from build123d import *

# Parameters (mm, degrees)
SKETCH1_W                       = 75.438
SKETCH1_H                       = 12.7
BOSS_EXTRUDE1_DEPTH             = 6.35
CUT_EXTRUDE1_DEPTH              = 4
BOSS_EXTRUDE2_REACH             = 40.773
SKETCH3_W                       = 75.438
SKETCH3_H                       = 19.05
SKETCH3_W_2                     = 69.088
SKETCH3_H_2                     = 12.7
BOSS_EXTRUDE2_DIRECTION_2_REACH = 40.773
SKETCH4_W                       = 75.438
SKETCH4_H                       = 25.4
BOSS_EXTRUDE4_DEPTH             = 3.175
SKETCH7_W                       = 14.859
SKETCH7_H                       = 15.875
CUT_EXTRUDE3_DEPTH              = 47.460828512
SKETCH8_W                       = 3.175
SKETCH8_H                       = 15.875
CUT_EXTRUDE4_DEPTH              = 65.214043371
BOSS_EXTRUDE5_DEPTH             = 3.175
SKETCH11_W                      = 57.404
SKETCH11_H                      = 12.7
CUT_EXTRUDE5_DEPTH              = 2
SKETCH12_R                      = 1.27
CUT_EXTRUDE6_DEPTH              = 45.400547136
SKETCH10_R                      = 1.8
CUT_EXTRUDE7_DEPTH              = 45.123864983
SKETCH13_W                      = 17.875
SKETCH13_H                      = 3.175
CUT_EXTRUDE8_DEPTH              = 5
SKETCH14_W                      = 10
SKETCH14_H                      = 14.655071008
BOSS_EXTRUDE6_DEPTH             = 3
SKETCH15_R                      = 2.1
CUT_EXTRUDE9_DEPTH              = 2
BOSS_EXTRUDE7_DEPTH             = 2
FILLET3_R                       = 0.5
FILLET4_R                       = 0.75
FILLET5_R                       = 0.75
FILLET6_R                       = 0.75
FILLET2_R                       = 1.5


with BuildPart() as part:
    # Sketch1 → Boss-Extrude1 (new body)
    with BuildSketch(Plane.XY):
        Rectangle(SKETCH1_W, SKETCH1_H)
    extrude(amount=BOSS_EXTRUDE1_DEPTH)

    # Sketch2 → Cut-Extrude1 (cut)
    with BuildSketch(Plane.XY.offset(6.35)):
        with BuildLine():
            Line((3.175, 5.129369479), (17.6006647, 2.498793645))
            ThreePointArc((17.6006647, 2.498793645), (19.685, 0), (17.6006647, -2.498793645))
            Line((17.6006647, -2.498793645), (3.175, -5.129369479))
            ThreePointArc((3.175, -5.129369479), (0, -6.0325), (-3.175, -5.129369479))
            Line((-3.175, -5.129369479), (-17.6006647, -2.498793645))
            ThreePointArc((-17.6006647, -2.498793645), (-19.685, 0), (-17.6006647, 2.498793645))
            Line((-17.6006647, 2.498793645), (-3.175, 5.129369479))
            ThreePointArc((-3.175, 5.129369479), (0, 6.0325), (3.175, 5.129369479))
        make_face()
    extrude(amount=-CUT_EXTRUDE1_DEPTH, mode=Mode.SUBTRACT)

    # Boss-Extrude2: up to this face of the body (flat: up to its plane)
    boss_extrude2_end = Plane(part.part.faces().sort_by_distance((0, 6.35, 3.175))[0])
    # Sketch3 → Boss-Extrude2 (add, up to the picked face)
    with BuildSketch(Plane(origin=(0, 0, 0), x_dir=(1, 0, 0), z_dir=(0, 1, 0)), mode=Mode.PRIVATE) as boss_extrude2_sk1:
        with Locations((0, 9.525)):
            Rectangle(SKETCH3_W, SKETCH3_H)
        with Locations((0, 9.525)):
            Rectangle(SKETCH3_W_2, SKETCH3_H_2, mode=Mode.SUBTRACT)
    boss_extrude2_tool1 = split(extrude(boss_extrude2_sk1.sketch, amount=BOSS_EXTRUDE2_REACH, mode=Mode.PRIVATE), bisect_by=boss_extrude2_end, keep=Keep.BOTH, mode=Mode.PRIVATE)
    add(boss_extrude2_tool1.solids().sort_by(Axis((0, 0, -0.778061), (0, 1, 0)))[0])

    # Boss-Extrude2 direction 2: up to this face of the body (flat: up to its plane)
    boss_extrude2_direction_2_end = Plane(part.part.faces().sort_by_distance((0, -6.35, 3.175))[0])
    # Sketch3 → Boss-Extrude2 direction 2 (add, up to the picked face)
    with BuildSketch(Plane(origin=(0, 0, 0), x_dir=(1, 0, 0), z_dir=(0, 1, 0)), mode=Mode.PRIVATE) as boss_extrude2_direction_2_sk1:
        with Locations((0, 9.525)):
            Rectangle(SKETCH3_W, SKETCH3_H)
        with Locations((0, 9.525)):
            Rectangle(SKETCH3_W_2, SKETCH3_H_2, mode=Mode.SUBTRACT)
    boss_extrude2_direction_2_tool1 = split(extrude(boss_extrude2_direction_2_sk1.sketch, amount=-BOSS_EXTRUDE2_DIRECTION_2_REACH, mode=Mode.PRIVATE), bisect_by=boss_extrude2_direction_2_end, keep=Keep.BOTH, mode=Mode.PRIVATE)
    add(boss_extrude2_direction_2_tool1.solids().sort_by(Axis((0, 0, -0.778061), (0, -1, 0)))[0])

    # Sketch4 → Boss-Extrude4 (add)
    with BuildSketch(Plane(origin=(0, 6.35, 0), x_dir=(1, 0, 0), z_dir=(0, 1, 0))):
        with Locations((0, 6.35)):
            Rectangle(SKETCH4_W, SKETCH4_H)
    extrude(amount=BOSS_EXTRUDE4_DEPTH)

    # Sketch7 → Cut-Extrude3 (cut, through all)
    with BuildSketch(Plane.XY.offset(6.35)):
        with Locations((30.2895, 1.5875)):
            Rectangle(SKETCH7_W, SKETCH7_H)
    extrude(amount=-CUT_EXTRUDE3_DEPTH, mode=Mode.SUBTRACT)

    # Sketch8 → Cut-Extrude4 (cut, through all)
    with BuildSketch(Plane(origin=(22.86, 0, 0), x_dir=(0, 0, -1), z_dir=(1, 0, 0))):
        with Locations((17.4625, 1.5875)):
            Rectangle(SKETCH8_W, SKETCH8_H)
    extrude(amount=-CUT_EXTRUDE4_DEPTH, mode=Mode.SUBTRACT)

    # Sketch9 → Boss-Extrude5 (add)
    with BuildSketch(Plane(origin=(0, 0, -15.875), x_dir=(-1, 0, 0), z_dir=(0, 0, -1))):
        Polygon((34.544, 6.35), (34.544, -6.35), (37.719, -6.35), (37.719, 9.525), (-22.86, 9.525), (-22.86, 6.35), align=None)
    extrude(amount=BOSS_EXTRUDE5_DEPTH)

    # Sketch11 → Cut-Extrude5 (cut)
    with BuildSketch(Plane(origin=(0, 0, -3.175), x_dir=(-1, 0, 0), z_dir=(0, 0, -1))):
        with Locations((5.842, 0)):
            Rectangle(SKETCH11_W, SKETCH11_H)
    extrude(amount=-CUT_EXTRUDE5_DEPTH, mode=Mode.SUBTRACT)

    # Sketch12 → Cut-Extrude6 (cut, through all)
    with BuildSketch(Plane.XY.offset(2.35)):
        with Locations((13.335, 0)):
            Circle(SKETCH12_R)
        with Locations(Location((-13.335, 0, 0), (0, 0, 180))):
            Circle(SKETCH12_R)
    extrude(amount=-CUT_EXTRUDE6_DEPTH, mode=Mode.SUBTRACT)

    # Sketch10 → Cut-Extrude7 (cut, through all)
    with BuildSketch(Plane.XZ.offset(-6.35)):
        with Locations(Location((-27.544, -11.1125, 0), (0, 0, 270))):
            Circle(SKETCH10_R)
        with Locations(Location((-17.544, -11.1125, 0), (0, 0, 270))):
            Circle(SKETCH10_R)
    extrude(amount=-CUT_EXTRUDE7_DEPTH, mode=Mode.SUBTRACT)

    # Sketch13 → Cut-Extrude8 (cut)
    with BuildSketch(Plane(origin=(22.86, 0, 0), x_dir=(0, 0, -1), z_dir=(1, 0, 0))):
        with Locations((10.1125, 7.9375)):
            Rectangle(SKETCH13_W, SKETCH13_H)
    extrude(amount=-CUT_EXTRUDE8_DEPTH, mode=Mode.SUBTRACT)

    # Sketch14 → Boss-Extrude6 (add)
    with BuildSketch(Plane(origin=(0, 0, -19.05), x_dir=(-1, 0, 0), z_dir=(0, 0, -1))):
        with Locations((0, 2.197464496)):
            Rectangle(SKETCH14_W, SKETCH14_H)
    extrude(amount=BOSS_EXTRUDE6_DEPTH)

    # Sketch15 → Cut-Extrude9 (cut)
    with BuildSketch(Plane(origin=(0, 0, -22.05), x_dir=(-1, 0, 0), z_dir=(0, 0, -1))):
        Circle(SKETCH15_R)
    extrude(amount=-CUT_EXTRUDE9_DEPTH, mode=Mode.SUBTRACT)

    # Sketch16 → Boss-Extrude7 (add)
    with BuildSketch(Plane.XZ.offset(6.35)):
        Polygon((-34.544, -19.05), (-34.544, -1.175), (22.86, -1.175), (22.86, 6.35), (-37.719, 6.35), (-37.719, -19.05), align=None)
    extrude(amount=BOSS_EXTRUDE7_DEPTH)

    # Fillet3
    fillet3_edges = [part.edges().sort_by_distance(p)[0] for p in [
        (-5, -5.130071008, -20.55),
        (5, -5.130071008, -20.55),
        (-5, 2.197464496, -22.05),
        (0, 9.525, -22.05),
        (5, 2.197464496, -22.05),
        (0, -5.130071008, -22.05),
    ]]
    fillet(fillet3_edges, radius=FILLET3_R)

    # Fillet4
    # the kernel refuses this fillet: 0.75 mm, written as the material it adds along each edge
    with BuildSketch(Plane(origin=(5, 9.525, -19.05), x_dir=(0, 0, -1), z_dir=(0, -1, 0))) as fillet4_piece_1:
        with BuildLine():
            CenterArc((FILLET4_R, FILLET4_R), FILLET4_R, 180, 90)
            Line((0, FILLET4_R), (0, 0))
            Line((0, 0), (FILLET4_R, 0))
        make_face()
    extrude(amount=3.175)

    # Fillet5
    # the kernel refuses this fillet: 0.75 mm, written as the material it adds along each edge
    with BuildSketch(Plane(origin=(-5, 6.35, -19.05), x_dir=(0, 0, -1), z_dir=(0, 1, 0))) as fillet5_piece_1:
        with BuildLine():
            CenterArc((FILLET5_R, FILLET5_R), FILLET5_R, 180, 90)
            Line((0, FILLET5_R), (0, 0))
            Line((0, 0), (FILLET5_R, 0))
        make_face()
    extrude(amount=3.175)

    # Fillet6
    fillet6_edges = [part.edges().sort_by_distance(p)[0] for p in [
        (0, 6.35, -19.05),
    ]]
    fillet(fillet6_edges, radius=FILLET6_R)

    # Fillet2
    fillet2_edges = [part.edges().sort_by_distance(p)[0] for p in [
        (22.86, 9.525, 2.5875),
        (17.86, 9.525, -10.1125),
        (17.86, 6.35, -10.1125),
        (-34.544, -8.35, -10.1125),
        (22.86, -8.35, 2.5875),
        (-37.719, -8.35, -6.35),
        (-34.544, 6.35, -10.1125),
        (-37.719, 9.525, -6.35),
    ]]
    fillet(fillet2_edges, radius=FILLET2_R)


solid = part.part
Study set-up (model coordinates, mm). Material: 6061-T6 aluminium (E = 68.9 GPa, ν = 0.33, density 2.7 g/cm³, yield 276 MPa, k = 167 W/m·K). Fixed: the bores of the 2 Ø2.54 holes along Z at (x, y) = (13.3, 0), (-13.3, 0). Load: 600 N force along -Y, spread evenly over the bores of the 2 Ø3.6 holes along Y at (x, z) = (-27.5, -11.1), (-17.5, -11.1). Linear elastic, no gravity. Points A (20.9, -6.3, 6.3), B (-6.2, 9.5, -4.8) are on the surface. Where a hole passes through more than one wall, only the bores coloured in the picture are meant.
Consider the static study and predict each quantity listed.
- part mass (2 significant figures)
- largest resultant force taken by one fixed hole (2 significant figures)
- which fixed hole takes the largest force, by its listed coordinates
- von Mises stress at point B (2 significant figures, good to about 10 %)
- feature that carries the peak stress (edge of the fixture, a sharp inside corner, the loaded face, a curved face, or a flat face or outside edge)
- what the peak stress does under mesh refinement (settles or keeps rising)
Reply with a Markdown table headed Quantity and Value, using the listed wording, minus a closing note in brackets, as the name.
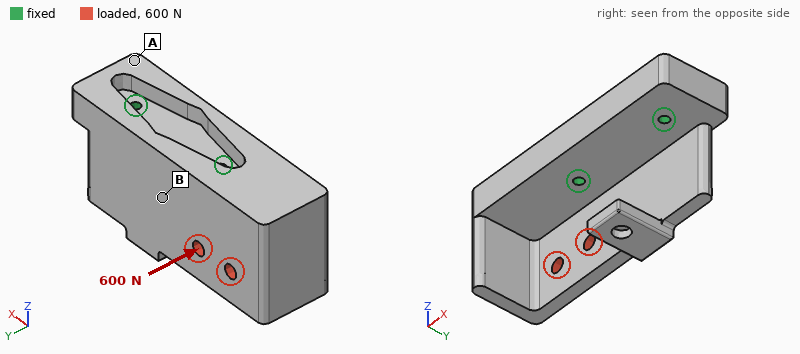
| Quantity | Value |
|---|---|
| part mass | 30 g |
| largest resultant force taken by one fixed hole | 780 N |
| which fixed hole takes the largest force, by its listed coordinates | (-13.3, 0) |
| von Mises stress at point B | 36 MPa |
| feature that carries the peak stress | edge of the fixture |
| what the peak stress does under mesh refinement | keeps rising |
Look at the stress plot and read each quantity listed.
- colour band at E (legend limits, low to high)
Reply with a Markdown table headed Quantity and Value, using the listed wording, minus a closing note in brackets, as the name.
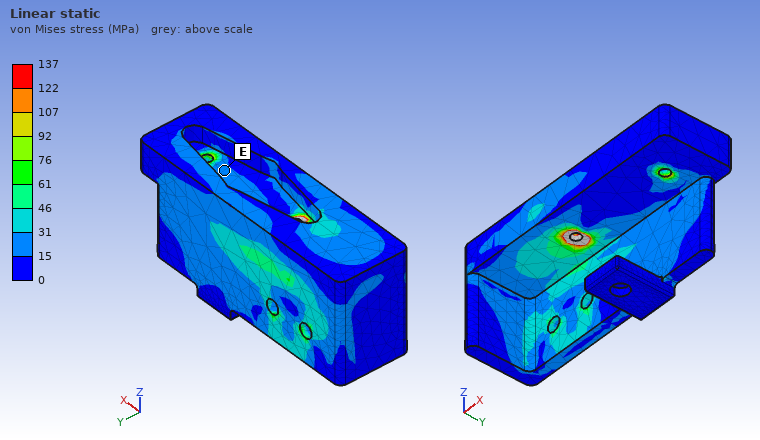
| Quantity | Value |
|---|---|
| colour band at E | 15 to 31 MPa |
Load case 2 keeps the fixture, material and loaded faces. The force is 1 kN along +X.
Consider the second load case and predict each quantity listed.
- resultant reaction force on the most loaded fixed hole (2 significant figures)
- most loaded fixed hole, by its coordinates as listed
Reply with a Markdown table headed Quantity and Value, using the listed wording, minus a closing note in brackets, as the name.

| Quantity | Value |
|---|---|
| resultant reaction force on the most loaded fixed hole | 780 N |
| most loaded fixed hole, by its coordinates as listed | (-13.3, 0) |
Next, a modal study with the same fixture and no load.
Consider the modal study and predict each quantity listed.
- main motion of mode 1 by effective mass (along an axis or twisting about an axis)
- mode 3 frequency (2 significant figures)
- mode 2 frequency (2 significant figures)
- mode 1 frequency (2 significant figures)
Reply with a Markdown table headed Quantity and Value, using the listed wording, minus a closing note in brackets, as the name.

| Quantity | Value |
|---|---|
| main motion of mode 1 by effective mass | along Y |
| mode 3 frequency | 6300 Hz |
| mode 2 frequency | 5100 Hz |
| mode 1 frequency | 3500 Hz |
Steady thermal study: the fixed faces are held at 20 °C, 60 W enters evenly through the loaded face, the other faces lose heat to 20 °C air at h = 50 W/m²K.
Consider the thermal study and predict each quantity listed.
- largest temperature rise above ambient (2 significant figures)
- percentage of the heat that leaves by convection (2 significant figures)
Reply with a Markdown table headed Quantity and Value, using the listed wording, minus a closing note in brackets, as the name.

| Quantity | Value |
|---|---|
| largest temperature rise above ambient | 70 K |
| percentage of the heat that leaves by convection | 13 % |
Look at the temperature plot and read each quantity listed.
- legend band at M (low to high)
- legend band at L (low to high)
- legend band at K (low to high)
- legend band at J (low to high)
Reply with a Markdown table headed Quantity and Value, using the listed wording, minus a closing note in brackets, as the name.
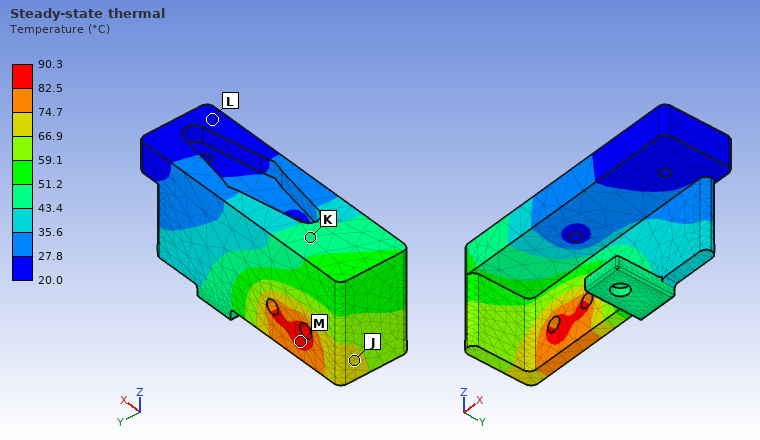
| Quantity | Value |
|---|---|
| legend band at M | 82.5 to 90.3 °C |
| legend band at L | 20.0 to 27.8 °C |
| legend band at K | 43.4 to 51.2 °C |
| legend band at J | 66.9 to 74.7 °C |
